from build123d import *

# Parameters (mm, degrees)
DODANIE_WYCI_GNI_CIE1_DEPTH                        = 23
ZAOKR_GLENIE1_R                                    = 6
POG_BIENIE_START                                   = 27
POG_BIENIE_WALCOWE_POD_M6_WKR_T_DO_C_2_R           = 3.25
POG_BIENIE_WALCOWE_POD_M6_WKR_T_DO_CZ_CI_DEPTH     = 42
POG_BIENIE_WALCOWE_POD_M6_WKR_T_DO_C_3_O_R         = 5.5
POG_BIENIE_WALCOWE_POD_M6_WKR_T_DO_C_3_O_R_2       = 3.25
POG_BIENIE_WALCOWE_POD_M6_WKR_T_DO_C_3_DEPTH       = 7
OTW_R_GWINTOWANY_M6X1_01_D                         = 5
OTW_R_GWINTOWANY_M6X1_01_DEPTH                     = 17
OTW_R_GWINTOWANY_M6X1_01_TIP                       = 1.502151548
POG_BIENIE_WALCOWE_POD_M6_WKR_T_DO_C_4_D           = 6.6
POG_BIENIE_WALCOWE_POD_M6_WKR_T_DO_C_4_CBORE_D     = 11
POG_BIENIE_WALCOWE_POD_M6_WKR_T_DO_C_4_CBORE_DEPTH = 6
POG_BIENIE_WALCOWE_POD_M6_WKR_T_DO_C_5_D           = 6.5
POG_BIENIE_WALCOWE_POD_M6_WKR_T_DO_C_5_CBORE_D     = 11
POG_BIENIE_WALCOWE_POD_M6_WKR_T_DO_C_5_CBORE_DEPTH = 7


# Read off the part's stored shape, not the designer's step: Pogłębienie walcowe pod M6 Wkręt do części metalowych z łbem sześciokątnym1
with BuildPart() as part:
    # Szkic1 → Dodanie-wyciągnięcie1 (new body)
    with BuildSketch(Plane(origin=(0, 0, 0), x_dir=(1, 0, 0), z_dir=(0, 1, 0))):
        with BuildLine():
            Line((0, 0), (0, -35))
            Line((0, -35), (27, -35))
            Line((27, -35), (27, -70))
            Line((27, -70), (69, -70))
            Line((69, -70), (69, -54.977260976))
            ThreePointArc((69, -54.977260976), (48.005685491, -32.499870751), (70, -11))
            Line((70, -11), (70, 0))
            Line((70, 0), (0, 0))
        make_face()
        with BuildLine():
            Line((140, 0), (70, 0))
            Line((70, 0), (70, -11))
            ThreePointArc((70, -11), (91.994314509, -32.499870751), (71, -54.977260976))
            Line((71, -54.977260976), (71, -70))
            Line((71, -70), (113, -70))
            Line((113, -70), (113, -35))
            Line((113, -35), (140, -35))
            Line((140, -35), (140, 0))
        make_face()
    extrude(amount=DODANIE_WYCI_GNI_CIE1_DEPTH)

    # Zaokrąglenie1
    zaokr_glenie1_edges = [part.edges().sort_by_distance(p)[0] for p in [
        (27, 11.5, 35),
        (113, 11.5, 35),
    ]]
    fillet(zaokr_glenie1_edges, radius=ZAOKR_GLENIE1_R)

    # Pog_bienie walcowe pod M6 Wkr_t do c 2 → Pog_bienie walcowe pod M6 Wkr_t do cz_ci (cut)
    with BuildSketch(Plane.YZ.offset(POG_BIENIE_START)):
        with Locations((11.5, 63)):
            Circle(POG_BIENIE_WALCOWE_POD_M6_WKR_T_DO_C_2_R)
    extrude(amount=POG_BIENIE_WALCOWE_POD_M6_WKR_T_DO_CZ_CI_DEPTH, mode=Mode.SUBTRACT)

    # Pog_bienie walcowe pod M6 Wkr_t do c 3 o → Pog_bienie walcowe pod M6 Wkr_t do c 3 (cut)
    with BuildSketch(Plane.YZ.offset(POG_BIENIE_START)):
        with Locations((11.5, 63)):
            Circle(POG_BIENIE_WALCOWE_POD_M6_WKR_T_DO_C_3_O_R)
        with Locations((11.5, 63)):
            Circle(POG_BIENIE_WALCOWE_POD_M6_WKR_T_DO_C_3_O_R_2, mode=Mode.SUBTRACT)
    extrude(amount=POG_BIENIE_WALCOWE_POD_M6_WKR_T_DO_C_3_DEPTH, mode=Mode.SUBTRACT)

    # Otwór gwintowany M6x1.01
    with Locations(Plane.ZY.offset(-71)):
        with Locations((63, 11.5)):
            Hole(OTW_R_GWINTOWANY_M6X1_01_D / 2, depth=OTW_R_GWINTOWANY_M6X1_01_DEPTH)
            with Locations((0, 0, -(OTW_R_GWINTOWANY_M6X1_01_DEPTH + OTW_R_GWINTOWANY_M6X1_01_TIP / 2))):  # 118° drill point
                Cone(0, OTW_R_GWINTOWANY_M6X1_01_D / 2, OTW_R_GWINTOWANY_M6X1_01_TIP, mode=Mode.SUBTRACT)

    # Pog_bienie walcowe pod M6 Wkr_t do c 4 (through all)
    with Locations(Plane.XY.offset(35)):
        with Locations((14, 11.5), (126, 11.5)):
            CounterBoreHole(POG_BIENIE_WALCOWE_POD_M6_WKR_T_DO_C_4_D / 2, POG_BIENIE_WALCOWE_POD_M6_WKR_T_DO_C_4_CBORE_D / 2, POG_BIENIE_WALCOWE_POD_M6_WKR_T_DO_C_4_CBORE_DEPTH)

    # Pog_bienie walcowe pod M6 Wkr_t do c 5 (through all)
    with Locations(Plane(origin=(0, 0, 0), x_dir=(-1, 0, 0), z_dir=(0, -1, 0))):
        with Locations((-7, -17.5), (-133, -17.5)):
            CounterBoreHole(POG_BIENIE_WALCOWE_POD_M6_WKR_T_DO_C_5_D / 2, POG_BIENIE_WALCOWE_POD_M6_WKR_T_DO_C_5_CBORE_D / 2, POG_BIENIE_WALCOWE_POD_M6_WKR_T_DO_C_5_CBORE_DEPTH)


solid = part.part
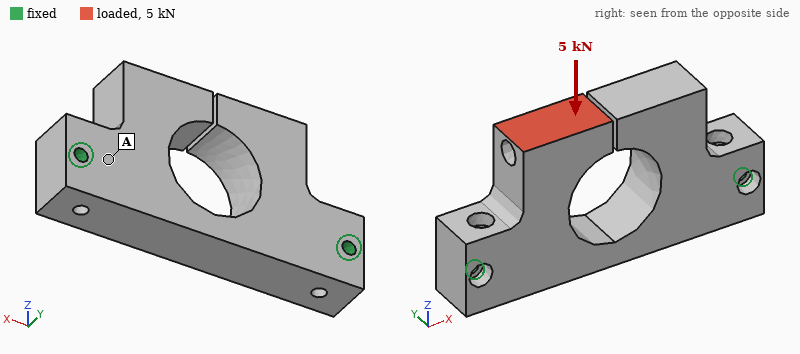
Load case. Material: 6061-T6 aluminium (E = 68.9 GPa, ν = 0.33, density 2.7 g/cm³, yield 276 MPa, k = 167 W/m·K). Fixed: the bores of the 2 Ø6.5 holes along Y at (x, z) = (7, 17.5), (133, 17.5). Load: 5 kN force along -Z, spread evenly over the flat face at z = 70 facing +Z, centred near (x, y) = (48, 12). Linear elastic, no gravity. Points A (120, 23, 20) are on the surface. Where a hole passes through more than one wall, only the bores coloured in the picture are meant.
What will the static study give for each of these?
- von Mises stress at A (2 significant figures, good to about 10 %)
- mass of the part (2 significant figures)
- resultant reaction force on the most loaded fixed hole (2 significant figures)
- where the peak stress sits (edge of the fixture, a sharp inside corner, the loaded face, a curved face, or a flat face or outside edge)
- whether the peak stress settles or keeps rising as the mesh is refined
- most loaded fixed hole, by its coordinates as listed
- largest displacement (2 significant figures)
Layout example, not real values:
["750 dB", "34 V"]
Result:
["13 MPa", "380 g", "5.2 kN", "edge of the fixture", "keeps rising", "(7, 17.5)", "0.17 mm"]
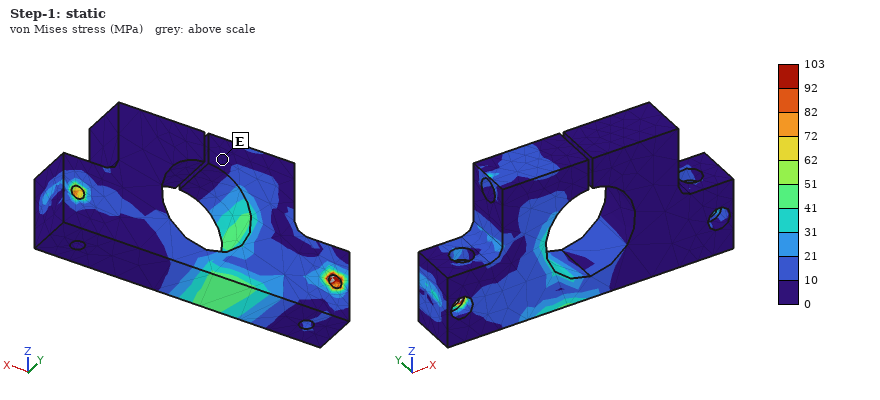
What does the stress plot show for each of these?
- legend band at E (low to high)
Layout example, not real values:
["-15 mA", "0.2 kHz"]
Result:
["0 to 10 MPa"]
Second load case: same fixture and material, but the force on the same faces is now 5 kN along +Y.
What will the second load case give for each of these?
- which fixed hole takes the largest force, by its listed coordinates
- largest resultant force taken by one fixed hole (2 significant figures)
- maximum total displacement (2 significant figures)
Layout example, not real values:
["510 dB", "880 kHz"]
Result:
["(7, 17.5)", "4.2 kN", "0.57 mm"]
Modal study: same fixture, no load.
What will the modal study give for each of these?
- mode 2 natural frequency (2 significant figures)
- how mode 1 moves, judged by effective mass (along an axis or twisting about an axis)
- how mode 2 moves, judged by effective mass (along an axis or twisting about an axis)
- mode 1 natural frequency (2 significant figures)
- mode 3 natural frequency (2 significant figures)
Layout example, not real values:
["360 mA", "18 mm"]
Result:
["2500 Hz", "along Y", "along Z", "2300 Hz", "2700 Hz"]
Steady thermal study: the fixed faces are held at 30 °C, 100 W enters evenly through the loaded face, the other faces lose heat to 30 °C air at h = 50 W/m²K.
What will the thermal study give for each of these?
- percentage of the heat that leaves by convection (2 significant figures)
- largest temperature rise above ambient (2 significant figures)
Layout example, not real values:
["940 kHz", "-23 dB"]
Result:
["20 %", "65 K"]
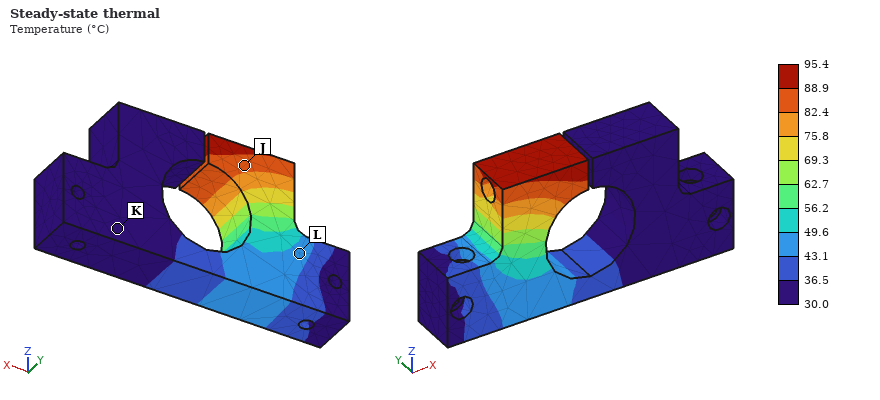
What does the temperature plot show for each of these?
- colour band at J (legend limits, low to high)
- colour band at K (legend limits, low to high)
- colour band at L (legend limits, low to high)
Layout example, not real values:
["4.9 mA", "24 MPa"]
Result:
["82.4 to 88.9 °C", "30.0 to 36.5 °C", "43.1 to 49.6 °C"]
